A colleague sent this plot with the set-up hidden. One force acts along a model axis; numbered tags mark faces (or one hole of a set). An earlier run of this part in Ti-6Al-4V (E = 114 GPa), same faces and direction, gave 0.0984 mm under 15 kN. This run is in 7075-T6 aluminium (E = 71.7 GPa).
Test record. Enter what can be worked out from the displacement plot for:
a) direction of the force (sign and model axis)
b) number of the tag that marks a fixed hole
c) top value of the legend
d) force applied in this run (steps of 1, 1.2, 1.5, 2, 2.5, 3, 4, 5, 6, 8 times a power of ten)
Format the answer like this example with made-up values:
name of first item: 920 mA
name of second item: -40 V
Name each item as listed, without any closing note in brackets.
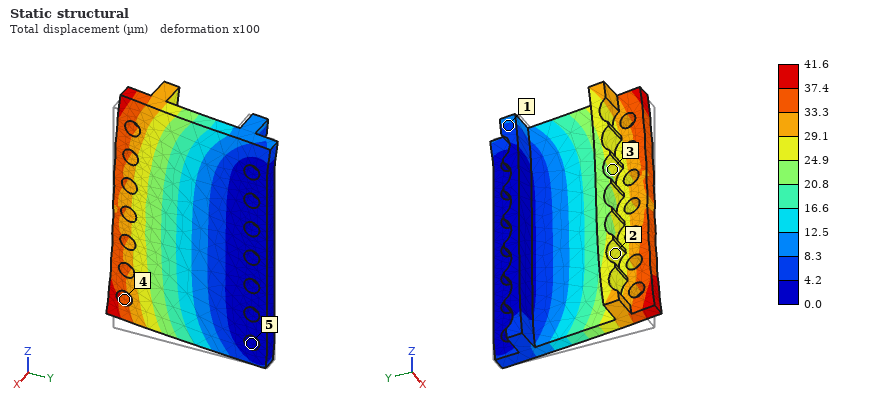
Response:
direction of the force: +Z
number of the tag that marks a fixed hole: 5
top value of the legend: 41.6 µm
force applied in this run: 4 kN
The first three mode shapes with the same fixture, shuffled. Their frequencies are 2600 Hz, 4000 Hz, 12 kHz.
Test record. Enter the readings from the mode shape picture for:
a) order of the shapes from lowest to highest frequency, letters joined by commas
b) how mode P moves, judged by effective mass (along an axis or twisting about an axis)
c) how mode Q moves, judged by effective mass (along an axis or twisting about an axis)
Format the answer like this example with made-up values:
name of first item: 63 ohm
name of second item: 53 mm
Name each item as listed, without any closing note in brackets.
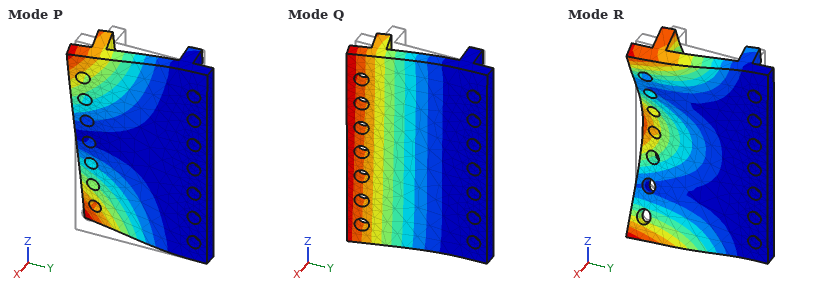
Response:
order of the shapes from lowest to highest frequency, letters joined by commas: Q, P, R
how mode P moves, judged by effective mass: twisting about Y
how mode Q moves, judged by effective mass: along X
